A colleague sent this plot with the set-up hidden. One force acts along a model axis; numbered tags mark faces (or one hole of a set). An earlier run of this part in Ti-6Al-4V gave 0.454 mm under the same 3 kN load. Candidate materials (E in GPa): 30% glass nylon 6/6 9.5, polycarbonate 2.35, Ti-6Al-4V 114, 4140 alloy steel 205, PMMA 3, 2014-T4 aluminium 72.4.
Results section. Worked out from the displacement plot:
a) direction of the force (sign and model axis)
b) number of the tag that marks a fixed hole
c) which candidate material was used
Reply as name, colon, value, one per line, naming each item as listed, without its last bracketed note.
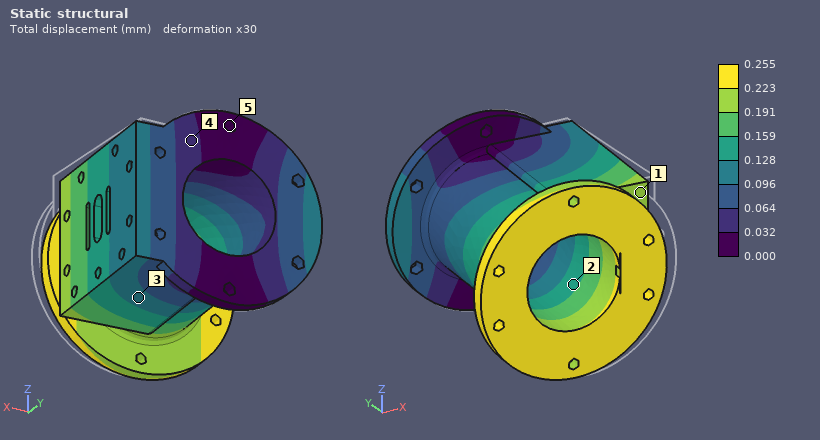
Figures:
direction of the force: -X
number of the tag that marks a fixed hole: 5
which candidate material was used: 4140 alloy steel
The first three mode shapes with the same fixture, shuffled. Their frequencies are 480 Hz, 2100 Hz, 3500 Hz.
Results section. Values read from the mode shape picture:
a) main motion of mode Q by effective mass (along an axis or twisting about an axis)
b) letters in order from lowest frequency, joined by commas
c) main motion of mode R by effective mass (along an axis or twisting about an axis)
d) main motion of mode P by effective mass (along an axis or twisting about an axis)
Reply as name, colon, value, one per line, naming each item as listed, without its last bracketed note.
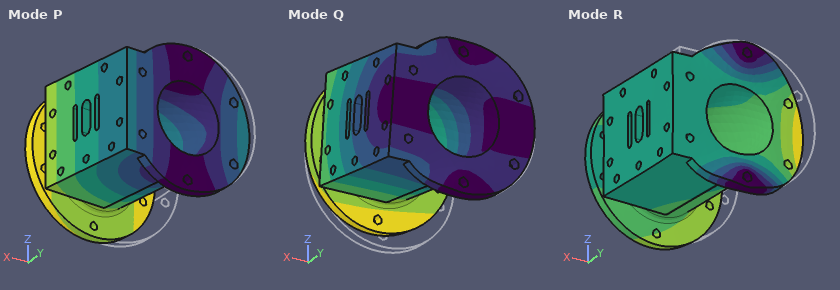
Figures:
main motion of mode Q by effective mass: along Z
letters in order from lowest frequency, joined by commas: P, Q, R
main motion of mode R by effective mass: along Y
main motion of mode P by effective mass: along X
